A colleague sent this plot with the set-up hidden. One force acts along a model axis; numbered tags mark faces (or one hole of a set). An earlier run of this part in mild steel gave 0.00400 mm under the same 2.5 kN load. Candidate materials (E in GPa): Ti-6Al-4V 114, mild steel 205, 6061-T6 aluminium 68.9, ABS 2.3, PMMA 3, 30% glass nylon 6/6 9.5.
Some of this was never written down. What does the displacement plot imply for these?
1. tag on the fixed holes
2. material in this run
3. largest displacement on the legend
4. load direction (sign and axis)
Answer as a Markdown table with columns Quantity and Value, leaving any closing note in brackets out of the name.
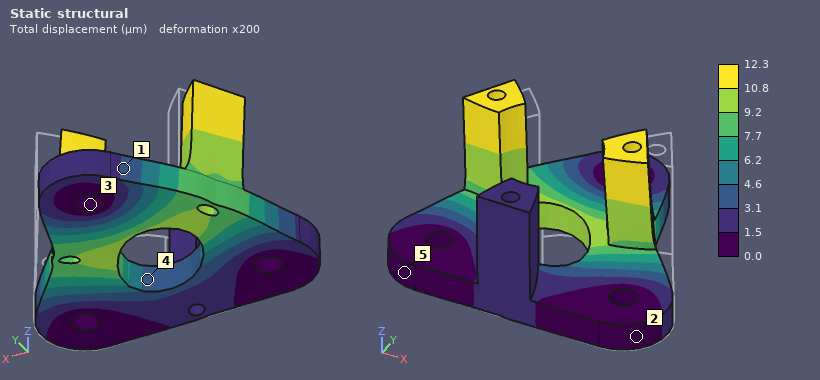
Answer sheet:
| Quantity | Value |
|---|---|
| tag on the fixed holes | 3 |
| material in this run | 6061-T6 aluminium |
| largest displacement on the legend | 12.3 µm |
| load direction | -X |
